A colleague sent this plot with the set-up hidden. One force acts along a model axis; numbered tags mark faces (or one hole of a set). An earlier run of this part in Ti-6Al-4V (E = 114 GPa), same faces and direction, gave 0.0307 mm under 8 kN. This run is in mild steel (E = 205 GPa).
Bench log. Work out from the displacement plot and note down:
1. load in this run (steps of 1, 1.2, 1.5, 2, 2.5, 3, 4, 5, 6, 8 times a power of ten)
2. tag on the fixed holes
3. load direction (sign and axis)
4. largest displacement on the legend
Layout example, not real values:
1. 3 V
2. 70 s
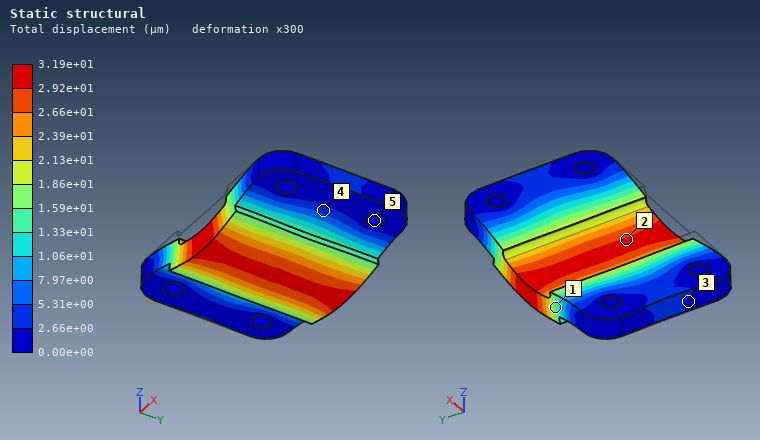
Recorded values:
1. 15 kN
2. 5
3. -Z
4. 3.19e+01 µm
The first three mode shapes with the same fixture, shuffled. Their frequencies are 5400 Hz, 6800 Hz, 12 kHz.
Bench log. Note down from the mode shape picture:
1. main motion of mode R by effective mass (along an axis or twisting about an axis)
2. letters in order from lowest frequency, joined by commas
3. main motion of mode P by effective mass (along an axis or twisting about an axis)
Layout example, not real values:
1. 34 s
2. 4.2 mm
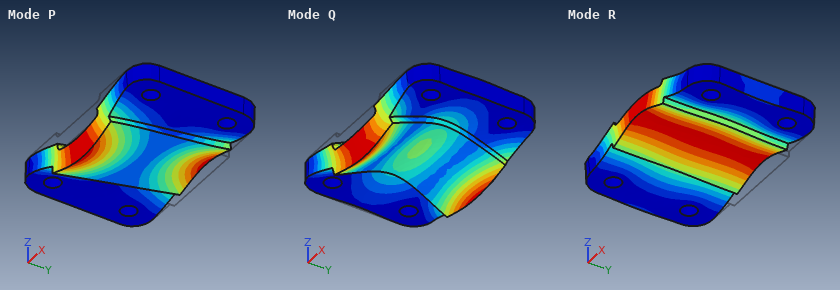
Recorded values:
1. along Z
2. R, P, Q
3. twisting about X
